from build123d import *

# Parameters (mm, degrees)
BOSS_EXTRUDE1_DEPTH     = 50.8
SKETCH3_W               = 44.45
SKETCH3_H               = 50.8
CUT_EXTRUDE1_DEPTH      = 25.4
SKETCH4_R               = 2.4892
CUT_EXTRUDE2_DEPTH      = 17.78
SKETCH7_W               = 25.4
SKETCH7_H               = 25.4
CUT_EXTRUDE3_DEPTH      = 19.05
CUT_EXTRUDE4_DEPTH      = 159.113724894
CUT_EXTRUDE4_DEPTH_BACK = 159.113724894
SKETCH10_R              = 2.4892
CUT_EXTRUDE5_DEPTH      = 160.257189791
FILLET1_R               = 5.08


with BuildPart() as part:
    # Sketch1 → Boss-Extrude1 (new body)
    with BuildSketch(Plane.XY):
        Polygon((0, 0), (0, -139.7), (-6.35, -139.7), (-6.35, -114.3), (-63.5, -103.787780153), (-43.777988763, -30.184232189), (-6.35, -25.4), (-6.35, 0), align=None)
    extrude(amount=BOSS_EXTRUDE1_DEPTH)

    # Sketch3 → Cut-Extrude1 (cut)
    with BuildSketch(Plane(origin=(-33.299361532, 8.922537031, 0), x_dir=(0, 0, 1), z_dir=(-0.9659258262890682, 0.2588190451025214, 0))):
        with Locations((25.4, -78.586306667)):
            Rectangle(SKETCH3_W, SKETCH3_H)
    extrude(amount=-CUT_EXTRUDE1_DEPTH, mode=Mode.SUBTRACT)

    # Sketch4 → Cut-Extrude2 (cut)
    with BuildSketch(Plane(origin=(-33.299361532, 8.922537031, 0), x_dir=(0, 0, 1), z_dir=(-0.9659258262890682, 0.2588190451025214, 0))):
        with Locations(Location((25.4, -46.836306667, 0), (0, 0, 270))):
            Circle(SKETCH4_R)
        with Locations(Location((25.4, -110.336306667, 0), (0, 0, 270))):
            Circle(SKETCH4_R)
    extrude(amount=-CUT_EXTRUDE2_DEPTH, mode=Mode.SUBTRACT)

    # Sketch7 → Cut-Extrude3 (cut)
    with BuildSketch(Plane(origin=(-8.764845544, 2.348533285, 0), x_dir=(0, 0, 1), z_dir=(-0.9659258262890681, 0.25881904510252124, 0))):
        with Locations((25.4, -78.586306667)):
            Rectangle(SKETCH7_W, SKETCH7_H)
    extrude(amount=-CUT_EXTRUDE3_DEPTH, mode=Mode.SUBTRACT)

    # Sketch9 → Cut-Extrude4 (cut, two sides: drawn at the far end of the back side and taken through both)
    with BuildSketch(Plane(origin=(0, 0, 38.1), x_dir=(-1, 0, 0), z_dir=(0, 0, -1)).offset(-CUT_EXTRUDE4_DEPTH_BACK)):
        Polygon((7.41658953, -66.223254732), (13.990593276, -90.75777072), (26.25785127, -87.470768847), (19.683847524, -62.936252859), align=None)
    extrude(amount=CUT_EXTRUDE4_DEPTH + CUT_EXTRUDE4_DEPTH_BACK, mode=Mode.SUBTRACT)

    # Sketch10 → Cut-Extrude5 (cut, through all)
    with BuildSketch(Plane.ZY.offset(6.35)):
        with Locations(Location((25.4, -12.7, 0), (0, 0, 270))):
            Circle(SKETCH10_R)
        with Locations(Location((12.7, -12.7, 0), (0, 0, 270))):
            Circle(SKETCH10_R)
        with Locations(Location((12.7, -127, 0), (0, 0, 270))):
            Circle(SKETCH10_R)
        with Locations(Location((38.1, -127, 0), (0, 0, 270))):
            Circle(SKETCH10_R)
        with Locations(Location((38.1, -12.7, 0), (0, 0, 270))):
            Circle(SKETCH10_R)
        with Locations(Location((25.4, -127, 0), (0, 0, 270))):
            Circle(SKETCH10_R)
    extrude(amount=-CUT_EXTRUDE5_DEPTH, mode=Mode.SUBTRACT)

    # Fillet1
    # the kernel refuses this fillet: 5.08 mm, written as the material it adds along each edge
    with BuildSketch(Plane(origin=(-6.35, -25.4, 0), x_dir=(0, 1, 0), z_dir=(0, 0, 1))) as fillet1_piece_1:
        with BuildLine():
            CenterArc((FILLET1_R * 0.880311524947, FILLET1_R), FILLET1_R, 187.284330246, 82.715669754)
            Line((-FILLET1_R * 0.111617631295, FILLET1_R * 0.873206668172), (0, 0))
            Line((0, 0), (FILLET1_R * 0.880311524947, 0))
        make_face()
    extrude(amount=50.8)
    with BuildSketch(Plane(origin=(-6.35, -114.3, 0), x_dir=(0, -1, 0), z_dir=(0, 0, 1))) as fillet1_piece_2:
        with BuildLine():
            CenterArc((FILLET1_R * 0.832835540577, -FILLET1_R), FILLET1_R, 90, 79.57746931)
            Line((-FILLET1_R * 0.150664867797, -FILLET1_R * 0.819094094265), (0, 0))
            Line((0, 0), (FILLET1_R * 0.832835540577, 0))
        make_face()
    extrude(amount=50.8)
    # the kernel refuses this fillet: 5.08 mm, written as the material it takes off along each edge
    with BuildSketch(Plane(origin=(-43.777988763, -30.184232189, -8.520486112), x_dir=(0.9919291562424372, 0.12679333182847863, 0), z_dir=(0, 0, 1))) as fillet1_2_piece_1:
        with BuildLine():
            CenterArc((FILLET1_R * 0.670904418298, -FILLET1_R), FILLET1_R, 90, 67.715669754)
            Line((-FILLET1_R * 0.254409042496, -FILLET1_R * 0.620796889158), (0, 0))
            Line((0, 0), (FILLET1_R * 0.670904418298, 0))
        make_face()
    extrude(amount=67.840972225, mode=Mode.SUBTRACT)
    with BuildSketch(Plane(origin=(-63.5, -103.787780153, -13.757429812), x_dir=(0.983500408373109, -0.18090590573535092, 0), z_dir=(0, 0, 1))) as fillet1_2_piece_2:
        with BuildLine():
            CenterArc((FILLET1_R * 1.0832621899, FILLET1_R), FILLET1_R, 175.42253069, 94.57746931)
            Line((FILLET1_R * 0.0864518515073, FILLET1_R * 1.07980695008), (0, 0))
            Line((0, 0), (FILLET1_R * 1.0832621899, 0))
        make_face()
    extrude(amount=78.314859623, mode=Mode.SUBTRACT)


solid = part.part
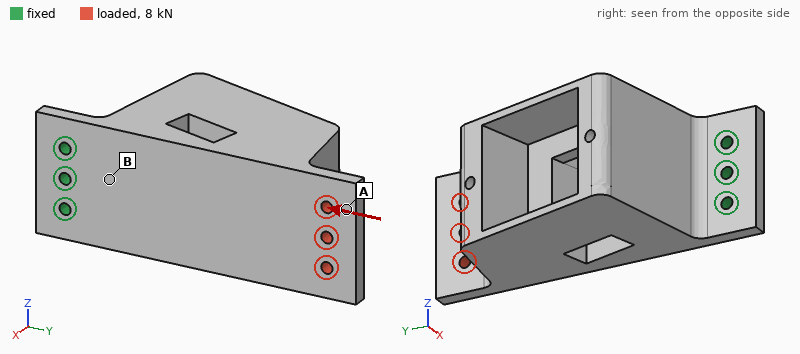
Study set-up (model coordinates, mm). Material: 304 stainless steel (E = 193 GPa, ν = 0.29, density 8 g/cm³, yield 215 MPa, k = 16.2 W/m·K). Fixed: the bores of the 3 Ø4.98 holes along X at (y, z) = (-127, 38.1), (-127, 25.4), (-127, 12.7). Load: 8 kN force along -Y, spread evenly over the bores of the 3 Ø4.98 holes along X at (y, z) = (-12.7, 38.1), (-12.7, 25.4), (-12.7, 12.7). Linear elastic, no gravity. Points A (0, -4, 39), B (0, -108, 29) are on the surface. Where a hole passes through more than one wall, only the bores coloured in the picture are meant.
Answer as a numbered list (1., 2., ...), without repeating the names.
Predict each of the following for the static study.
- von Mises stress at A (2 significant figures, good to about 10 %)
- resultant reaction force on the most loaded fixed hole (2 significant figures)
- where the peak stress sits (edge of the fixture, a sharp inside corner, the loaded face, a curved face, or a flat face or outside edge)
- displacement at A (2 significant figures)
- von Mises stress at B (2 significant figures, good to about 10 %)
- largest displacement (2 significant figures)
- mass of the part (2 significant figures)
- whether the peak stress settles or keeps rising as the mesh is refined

1. 8.5 MPa
2. 3.0 kN
3. edge of the fixture
4. 43 µm
5. 29 MPa
6. 46 µm
7. 1.3 kg
8. keeps rising
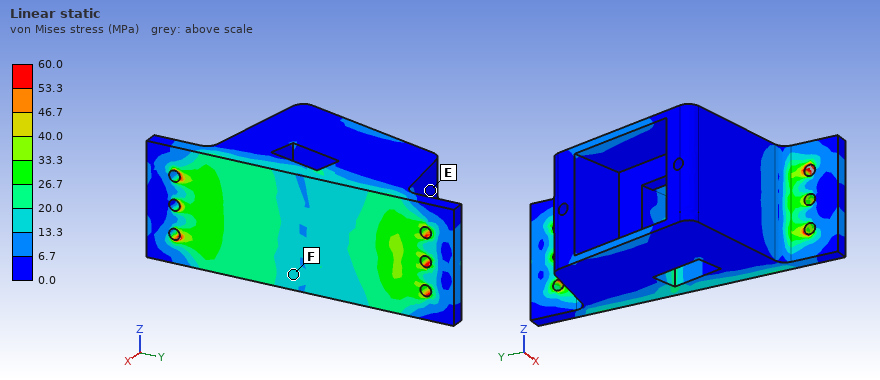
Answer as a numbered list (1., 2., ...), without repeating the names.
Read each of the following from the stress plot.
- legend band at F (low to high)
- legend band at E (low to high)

1. 13.3 to 20.0 MPa
2. 0.0 to 6.7 MPa
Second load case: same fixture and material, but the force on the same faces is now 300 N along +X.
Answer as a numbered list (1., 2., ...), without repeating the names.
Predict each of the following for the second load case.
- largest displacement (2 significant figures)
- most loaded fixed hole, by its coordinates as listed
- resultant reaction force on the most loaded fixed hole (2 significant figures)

1. 0.26 mm
2. (-127, 25.4)
3. 240 N
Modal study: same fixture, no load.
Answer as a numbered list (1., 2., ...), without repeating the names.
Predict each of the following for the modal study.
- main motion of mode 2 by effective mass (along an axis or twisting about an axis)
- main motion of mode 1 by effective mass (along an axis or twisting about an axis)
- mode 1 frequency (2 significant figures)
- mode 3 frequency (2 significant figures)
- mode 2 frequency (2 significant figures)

1. along Z
2. along X
3. 280 Hz
4. 1700 Hz
5. 1200 Hz
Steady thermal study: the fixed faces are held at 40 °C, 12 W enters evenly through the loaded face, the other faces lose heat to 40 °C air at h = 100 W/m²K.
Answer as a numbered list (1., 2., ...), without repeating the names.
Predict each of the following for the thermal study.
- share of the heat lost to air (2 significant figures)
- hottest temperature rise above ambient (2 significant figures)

1. 99 %
2. 34 K
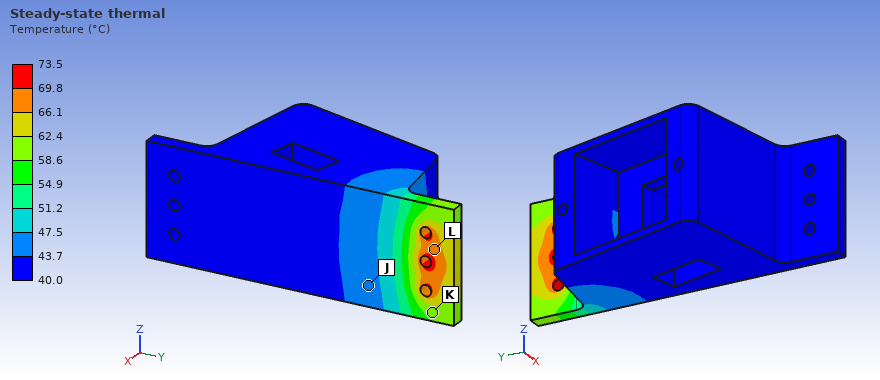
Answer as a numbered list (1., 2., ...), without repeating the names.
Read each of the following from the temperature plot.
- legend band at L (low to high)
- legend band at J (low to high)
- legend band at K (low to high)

1. 66.1 to 69.8 °C
2. 43.7 to 47.5 °C
3. 58.6 to 62.4 °C
